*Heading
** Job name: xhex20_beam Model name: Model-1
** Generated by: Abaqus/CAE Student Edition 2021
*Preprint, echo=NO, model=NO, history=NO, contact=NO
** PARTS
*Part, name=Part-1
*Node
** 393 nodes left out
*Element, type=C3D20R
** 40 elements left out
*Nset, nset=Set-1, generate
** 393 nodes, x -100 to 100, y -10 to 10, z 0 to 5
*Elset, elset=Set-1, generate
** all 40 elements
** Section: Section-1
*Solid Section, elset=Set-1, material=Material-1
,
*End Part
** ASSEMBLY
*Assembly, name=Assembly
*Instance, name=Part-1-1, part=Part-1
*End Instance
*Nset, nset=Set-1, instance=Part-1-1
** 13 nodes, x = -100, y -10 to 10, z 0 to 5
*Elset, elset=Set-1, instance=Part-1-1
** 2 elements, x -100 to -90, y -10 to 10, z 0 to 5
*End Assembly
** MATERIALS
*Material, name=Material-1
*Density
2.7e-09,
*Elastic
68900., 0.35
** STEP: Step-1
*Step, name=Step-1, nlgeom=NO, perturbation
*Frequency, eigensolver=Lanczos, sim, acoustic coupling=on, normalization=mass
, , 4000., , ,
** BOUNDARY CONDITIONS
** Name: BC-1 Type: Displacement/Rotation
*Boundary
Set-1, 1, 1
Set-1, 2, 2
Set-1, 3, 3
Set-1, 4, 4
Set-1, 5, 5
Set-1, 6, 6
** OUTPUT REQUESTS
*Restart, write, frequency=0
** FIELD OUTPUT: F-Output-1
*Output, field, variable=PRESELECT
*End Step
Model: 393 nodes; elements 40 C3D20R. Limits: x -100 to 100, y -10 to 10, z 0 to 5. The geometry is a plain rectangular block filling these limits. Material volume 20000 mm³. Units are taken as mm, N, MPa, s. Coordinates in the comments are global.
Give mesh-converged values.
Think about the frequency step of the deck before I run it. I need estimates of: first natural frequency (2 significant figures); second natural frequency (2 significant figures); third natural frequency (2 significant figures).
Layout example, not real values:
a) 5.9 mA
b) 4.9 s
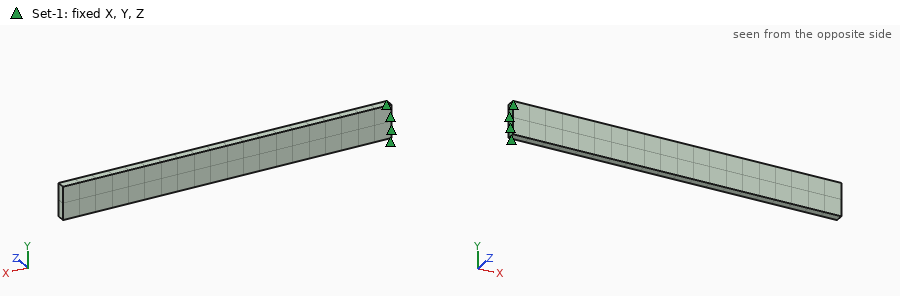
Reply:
a) 100 Hz
b) 410 Hz
c) 640 Hz
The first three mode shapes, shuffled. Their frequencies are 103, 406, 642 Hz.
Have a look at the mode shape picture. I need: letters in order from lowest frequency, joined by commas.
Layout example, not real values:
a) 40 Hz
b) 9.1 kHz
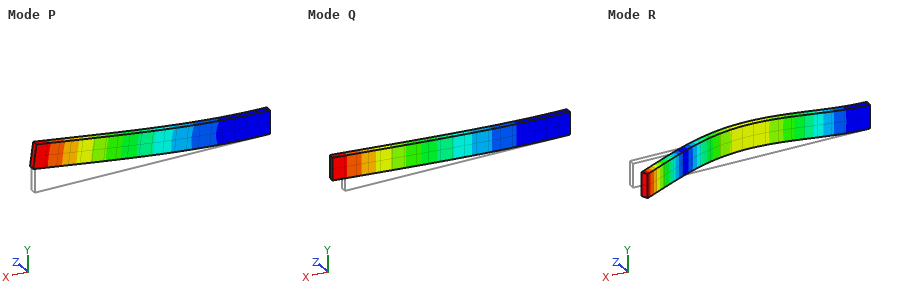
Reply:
a) Q, P, R
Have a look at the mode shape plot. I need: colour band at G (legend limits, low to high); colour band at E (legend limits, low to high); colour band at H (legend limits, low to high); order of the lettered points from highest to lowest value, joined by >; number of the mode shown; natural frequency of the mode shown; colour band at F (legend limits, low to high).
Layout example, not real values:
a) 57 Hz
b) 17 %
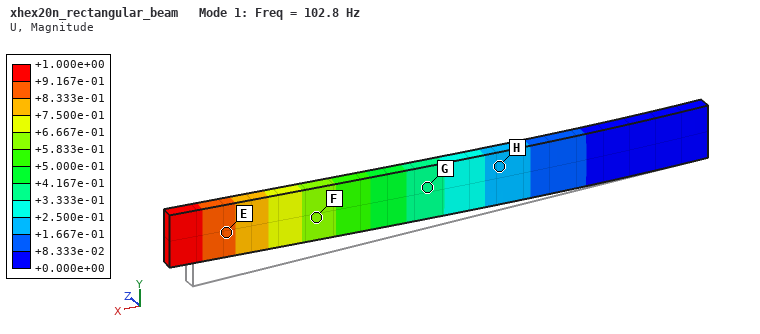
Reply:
a) +3.333e-01 to +4.167e-01
b) +8.333e-01 to +9.167e-01
c) +1.667e-01 to +2.500e-01
d) E > F > G > H
e) 1
f) 102.8 Hz
g) +5.833e-01 to +6.667e-01
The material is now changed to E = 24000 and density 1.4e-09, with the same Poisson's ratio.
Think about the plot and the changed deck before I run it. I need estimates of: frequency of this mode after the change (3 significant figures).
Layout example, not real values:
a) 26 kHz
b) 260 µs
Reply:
a) 84.3 Hz
